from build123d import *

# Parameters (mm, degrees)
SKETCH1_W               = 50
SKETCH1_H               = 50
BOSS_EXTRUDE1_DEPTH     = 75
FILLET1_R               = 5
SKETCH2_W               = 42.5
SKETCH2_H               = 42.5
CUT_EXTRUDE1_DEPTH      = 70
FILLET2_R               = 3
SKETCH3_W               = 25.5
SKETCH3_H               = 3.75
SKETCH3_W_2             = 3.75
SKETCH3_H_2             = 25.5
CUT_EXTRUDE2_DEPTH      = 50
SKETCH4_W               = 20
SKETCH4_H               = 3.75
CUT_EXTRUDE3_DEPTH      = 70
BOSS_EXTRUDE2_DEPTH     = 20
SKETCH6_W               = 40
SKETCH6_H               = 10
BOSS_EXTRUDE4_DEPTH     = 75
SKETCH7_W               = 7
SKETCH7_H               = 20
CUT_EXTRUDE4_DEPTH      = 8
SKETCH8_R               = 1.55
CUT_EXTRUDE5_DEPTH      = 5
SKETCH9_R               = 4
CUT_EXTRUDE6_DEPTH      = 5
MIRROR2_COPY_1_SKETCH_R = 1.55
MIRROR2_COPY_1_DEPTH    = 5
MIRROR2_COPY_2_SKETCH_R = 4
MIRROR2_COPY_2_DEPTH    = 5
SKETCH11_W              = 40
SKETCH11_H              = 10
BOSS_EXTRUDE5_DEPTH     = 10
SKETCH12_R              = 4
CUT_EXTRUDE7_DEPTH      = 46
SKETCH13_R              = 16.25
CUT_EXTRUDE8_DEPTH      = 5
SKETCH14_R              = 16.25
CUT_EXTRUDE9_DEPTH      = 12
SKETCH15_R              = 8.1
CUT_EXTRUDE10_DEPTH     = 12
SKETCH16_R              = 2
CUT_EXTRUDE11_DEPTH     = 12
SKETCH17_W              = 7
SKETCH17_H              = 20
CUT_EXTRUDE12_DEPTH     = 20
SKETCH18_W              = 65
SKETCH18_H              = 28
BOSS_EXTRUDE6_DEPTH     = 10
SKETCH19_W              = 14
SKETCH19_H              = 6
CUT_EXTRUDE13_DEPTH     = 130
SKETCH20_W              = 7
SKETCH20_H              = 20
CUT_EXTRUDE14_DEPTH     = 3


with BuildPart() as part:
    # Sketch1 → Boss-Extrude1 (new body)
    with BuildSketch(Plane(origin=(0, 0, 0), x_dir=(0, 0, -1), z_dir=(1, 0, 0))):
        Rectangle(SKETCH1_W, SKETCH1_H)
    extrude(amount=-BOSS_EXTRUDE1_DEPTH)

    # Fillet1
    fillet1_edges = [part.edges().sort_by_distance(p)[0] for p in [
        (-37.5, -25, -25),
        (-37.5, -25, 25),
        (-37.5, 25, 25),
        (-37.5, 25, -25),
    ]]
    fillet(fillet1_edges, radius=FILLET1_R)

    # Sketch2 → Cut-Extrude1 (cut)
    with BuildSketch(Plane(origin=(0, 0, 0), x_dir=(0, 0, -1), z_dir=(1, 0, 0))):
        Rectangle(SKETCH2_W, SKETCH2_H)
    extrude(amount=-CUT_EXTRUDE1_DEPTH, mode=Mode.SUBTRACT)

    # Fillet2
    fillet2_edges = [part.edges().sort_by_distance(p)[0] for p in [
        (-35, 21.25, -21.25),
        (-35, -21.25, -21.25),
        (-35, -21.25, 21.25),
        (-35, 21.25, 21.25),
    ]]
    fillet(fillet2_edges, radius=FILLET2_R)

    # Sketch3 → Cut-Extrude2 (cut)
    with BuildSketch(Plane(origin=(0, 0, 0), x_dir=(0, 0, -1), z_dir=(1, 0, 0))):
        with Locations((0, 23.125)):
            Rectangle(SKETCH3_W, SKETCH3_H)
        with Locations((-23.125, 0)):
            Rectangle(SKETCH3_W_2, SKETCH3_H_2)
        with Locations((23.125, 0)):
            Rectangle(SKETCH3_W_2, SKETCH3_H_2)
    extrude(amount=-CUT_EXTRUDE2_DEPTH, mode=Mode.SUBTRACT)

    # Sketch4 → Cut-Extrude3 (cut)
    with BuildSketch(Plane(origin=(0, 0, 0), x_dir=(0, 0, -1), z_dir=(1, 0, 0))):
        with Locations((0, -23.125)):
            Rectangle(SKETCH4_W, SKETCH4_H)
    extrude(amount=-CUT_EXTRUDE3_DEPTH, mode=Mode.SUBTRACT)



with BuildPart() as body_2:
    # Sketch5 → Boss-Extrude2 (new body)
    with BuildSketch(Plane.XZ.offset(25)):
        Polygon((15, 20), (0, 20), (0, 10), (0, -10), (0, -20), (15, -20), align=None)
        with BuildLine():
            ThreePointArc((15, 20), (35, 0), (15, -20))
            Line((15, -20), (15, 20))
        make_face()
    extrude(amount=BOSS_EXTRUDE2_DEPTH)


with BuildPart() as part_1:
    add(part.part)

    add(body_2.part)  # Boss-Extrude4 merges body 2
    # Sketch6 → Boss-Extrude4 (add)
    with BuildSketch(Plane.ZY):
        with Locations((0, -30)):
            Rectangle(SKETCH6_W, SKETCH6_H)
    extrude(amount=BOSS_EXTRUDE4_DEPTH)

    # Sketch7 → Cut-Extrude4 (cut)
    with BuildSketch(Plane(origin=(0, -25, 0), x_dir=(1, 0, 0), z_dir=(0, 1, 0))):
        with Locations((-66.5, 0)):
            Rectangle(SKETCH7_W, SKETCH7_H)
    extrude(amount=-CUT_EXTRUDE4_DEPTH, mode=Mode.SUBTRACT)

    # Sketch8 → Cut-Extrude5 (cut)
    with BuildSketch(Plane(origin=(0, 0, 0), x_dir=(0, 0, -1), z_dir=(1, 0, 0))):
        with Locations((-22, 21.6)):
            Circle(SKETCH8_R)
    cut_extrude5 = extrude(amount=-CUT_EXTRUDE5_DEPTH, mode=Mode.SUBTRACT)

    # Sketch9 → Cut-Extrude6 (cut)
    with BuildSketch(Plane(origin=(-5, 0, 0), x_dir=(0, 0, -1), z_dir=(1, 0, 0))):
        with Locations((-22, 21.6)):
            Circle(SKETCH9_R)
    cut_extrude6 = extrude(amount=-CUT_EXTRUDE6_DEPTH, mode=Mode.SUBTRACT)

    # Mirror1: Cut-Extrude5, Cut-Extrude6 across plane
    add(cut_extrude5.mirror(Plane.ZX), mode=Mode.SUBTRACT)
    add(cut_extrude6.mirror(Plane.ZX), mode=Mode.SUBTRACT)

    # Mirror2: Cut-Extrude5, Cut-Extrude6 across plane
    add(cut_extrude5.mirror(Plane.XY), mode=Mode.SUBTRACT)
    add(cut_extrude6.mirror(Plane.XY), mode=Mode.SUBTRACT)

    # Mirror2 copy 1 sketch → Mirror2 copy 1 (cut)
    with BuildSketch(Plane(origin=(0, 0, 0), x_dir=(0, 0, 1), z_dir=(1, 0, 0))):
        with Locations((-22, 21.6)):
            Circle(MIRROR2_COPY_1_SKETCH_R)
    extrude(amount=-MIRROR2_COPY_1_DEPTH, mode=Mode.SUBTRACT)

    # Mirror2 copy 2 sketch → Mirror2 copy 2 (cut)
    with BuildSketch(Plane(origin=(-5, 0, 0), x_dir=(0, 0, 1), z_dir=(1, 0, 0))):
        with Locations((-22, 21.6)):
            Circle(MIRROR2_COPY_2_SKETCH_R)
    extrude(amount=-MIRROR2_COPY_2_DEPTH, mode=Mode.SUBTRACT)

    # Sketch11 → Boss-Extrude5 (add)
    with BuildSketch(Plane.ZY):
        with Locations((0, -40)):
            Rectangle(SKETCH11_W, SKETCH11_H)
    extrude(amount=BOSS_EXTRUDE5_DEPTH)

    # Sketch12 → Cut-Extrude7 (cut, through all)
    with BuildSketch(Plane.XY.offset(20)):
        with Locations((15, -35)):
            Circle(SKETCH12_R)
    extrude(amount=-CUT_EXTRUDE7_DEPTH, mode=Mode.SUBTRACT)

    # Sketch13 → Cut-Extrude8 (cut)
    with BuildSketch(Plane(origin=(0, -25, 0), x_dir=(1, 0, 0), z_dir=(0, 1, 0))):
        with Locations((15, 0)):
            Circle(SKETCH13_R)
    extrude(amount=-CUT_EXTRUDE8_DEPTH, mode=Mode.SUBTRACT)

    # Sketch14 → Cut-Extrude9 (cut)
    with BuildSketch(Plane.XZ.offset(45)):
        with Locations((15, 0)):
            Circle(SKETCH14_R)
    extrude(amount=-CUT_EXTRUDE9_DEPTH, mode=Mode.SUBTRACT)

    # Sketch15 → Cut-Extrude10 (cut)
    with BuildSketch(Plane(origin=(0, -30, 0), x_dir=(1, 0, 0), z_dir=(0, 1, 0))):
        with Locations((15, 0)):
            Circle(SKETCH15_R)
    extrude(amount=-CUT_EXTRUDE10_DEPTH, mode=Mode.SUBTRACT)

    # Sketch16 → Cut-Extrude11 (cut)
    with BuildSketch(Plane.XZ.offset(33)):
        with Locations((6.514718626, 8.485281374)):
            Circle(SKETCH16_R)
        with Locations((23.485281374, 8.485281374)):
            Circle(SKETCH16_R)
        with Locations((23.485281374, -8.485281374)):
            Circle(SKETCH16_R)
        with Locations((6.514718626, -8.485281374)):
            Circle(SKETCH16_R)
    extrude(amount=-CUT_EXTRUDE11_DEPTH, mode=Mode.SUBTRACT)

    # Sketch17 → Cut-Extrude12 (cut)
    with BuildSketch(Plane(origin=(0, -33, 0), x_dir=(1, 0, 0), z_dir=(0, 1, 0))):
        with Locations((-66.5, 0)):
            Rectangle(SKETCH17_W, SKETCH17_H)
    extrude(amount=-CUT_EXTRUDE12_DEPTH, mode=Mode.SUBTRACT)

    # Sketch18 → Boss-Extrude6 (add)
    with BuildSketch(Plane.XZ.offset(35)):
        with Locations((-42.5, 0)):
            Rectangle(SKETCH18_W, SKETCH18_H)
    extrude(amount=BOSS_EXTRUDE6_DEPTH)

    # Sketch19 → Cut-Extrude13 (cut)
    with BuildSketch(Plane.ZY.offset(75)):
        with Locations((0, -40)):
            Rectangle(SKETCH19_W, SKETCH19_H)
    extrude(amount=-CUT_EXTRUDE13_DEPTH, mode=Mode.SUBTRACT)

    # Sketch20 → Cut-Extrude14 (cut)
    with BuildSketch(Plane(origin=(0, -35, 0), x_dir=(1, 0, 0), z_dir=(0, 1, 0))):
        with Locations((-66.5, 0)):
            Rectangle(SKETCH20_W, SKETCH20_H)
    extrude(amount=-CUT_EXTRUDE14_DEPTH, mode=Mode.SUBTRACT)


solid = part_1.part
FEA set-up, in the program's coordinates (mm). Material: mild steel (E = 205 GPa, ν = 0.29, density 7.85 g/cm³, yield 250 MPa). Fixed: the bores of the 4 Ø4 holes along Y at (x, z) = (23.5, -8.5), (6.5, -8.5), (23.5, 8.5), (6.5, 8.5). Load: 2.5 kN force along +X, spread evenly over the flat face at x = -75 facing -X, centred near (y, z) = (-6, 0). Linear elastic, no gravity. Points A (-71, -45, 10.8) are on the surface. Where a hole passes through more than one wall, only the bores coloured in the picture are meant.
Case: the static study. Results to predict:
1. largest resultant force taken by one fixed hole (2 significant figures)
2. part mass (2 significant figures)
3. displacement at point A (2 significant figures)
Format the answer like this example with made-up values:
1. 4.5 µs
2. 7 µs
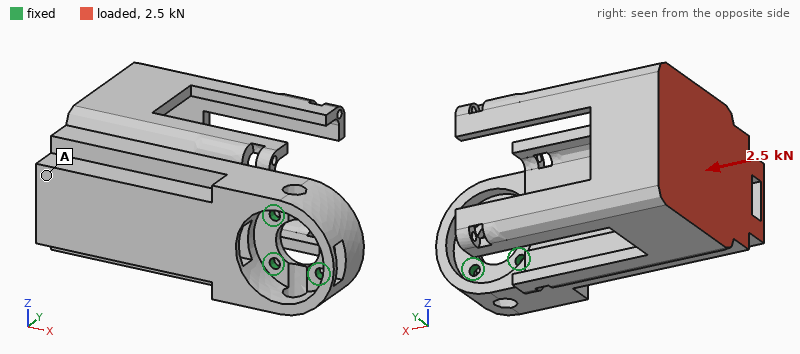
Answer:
1. 1.8 kN
2. 730 g
3. 0.15 mm
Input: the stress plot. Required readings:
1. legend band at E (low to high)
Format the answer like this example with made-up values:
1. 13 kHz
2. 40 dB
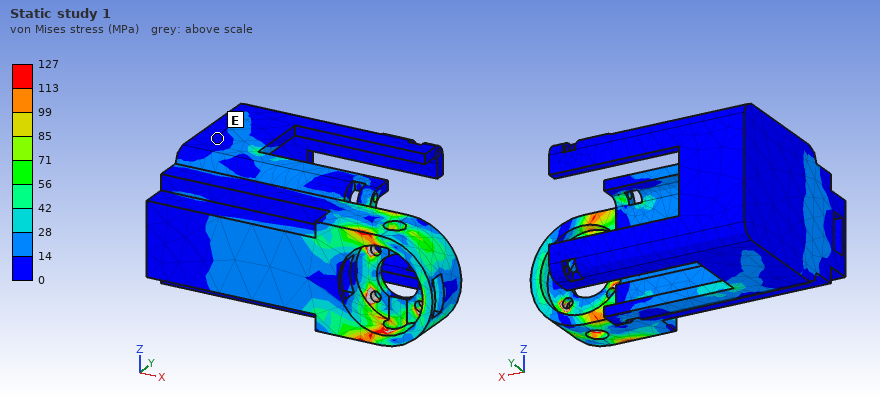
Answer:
1. 0 to 14 MPa
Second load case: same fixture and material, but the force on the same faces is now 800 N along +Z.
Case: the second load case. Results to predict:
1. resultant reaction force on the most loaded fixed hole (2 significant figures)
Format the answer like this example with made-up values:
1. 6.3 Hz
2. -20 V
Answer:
1. 2.1 kN
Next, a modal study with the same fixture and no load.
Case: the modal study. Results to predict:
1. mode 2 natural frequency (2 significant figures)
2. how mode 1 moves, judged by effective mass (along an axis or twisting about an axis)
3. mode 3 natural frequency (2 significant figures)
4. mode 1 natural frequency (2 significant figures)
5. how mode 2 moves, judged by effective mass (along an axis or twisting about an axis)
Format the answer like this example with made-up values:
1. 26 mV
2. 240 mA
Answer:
1. 910 Hz
2. along Y
3. 1600 Hz
4. 600 Hz
5. along Z
